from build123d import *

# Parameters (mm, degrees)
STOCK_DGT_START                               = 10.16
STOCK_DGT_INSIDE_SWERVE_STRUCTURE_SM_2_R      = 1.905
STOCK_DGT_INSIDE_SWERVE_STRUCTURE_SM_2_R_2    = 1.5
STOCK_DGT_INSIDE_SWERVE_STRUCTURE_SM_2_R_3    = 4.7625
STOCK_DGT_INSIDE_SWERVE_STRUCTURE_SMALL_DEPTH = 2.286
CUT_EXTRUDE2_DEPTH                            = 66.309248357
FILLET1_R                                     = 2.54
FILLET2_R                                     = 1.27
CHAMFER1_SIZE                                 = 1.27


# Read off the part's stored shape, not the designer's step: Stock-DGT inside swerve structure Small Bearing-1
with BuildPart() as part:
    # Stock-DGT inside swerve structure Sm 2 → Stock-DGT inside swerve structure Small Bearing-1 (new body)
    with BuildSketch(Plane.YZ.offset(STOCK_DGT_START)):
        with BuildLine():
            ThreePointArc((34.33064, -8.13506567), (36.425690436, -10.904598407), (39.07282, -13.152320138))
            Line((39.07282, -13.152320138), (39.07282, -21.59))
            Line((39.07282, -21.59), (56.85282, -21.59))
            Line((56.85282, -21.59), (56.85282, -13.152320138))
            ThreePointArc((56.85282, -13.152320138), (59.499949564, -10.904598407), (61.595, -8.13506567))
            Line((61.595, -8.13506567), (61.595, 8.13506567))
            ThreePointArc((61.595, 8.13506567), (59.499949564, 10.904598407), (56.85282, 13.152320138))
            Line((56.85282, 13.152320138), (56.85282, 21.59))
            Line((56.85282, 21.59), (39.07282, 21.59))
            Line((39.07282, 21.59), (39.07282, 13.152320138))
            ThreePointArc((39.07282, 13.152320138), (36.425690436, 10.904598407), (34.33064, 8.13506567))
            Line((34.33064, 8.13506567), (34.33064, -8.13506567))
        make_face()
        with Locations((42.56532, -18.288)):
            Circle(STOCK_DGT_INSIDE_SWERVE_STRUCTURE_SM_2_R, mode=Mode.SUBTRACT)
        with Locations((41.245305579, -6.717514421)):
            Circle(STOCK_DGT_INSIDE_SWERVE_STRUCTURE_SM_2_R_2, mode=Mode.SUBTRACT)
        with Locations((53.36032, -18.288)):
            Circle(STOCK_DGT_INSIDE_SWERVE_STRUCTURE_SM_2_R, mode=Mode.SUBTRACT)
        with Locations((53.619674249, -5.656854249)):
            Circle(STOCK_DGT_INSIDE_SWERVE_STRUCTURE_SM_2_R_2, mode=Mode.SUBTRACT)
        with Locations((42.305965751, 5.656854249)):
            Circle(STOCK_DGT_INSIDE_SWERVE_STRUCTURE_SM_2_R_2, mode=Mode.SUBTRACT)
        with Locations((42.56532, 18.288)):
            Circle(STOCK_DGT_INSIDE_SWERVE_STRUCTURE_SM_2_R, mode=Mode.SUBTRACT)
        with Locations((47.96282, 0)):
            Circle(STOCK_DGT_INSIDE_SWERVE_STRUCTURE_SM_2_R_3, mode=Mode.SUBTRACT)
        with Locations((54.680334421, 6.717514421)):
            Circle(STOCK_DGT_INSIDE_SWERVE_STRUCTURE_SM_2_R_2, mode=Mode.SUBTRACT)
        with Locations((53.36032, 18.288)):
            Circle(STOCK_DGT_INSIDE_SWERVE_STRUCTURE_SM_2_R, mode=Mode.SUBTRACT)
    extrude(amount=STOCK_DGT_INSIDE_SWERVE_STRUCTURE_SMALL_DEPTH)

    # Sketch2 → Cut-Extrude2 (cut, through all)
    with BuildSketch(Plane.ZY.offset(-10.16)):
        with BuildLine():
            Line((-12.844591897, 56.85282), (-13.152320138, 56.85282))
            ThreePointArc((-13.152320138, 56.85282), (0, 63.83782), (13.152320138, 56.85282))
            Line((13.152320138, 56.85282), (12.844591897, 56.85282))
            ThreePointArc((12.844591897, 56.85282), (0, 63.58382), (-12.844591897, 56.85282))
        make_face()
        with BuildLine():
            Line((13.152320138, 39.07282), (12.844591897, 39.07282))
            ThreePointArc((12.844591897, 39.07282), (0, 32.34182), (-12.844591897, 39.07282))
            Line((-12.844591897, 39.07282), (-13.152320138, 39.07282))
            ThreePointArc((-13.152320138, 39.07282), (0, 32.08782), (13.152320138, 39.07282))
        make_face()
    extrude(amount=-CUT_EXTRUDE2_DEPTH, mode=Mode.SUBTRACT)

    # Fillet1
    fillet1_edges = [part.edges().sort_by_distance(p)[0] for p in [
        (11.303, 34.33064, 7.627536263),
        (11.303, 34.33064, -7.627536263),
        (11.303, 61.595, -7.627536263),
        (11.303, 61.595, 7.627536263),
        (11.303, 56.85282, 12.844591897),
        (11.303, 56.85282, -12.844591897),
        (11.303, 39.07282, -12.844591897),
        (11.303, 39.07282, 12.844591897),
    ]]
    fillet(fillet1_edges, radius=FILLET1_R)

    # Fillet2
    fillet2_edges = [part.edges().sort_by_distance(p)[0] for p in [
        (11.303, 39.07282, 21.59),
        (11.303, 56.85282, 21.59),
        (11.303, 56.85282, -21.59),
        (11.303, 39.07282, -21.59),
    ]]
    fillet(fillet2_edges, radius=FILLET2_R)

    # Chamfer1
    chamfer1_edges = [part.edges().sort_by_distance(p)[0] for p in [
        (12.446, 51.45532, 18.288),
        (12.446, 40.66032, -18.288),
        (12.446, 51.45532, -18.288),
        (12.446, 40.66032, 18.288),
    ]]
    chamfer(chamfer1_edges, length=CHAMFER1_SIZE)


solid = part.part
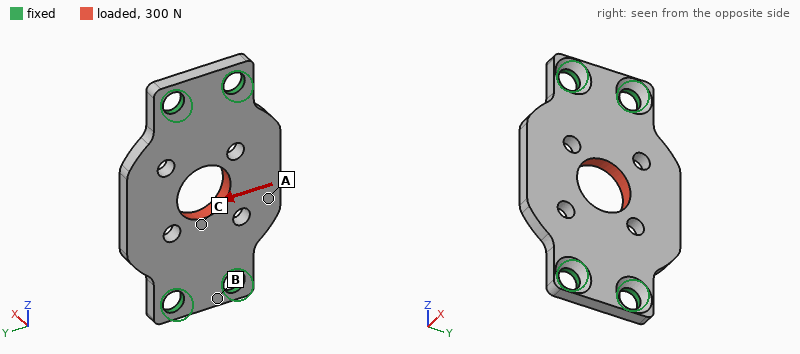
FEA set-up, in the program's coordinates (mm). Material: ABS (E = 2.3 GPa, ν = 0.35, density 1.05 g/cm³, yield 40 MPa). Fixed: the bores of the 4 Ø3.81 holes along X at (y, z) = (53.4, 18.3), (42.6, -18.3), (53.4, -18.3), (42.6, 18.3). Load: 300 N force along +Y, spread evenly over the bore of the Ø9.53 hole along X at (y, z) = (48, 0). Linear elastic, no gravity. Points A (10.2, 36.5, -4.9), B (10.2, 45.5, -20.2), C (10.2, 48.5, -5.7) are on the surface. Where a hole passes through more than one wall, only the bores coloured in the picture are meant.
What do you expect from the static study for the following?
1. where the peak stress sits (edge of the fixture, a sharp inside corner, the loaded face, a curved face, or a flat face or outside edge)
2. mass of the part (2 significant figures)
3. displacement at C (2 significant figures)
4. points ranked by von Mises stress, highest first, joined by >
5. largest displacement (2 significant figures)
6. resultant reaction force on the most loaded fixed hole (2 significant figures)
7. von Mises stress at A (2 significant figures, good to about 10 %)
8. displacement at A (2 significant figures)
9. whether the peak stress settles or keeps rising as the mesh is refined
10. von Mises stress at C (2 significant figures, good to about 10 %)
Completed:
edge of the fixture
1.9 g
71 µm
C > A > B
86 µm
93 N
5.4 MPa
69 µm
keeps rising
8.7 MPa
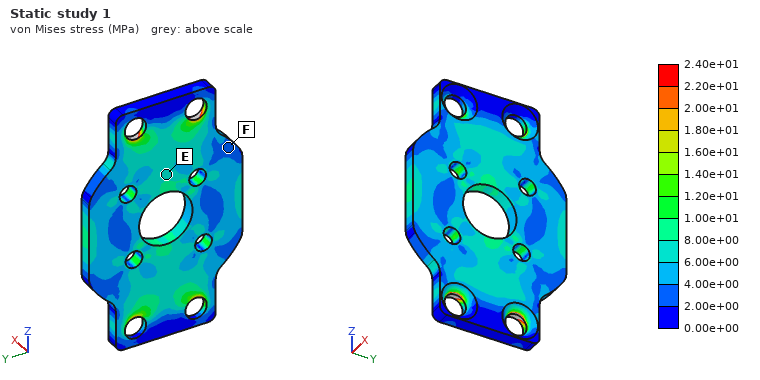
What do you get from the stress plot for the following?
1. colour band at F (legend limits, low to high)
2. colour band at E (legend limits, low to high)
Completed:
2.00e+00 to 4.00e+00 MPa
6.00e+00 to 8.00e+00 MPa
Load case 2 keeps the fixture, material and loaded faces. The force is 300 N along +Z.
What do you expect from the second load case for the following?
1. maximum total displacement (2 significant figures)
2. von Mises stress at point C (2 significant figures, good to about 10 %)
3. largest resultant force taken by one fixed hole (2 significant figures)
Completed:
42 µm
4.2 MPa
76 N
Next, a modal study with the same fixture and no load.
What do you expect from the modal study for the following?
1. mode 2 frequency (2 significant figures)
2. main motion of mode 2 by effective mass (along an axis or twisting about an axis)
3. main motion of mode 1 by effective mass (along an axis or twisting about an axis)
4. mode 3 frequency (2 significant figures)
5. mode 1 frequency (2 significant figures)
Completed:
2400 Hz
twisting about Z
along X
5600 Hz
2100 Hz
